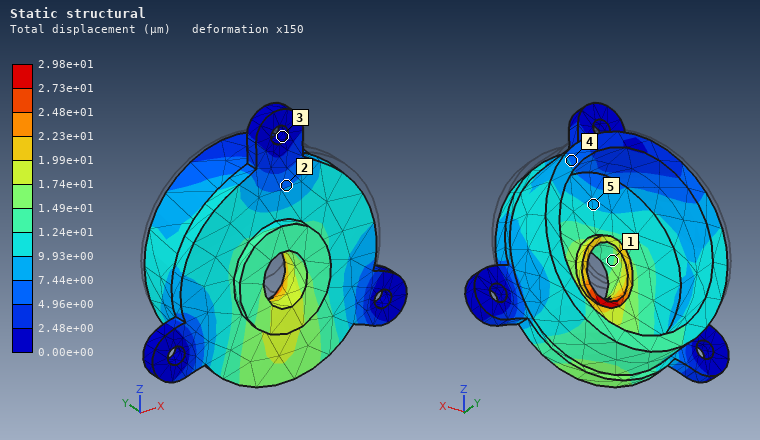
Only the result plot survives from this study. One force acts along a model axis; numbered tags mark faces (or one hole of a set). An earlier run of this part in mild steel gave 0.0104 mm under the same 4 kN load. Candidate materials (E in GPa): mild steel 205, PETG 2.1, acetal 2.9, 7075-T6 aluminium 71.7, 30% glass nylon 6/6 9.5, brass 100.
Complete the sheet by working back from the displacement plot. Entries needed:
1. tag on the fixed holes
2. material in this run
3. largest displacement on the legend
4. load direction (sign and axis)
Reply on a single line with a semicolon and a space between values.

3; 7075-T6 aluminium; 2.98e+01 µm; -Z
